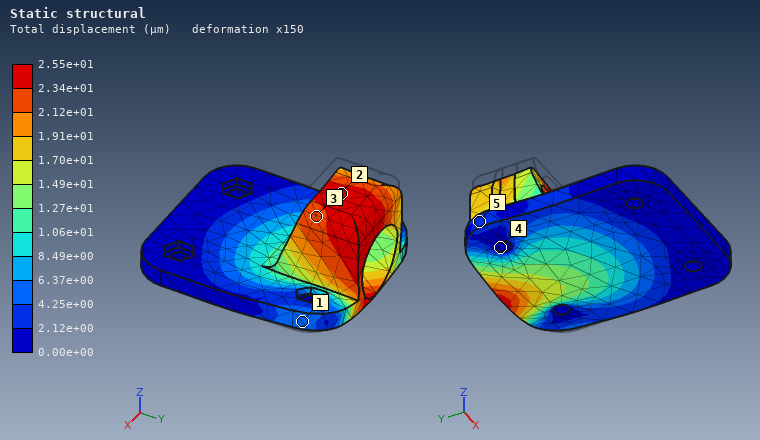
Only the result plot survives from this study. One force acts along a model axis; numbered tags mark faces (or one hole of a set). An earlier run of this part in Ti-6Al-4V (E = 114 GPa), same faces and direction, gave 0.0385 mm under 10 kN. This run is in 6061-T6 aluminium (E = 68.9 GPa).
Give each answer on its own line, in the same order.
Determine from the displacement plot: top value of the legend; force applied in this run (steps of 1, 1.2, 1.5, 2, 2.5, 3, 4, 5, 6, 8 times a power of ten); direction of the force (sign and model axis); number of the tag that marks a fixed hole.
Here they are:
2.55e+01 µm
4 kN
-Z
4
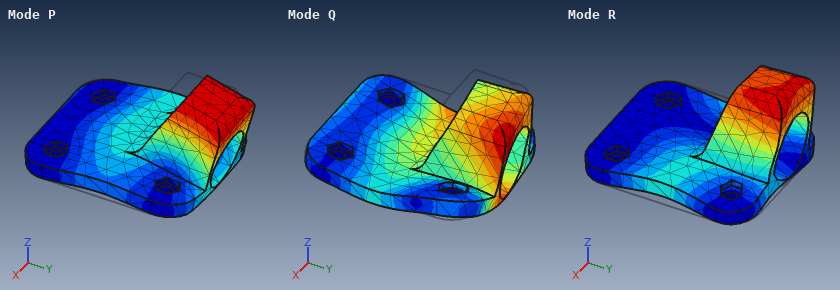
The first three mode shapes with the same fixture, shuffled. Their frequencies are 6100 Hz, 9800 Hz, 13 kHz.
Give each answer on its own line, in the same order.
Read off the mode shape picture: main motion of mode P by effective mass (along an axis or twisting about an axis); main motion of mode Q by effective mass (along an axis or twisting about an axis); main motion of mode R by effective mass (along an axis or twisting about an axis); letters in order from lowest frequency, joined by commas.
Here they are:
along Y
along Z
along X
P, R, Q
